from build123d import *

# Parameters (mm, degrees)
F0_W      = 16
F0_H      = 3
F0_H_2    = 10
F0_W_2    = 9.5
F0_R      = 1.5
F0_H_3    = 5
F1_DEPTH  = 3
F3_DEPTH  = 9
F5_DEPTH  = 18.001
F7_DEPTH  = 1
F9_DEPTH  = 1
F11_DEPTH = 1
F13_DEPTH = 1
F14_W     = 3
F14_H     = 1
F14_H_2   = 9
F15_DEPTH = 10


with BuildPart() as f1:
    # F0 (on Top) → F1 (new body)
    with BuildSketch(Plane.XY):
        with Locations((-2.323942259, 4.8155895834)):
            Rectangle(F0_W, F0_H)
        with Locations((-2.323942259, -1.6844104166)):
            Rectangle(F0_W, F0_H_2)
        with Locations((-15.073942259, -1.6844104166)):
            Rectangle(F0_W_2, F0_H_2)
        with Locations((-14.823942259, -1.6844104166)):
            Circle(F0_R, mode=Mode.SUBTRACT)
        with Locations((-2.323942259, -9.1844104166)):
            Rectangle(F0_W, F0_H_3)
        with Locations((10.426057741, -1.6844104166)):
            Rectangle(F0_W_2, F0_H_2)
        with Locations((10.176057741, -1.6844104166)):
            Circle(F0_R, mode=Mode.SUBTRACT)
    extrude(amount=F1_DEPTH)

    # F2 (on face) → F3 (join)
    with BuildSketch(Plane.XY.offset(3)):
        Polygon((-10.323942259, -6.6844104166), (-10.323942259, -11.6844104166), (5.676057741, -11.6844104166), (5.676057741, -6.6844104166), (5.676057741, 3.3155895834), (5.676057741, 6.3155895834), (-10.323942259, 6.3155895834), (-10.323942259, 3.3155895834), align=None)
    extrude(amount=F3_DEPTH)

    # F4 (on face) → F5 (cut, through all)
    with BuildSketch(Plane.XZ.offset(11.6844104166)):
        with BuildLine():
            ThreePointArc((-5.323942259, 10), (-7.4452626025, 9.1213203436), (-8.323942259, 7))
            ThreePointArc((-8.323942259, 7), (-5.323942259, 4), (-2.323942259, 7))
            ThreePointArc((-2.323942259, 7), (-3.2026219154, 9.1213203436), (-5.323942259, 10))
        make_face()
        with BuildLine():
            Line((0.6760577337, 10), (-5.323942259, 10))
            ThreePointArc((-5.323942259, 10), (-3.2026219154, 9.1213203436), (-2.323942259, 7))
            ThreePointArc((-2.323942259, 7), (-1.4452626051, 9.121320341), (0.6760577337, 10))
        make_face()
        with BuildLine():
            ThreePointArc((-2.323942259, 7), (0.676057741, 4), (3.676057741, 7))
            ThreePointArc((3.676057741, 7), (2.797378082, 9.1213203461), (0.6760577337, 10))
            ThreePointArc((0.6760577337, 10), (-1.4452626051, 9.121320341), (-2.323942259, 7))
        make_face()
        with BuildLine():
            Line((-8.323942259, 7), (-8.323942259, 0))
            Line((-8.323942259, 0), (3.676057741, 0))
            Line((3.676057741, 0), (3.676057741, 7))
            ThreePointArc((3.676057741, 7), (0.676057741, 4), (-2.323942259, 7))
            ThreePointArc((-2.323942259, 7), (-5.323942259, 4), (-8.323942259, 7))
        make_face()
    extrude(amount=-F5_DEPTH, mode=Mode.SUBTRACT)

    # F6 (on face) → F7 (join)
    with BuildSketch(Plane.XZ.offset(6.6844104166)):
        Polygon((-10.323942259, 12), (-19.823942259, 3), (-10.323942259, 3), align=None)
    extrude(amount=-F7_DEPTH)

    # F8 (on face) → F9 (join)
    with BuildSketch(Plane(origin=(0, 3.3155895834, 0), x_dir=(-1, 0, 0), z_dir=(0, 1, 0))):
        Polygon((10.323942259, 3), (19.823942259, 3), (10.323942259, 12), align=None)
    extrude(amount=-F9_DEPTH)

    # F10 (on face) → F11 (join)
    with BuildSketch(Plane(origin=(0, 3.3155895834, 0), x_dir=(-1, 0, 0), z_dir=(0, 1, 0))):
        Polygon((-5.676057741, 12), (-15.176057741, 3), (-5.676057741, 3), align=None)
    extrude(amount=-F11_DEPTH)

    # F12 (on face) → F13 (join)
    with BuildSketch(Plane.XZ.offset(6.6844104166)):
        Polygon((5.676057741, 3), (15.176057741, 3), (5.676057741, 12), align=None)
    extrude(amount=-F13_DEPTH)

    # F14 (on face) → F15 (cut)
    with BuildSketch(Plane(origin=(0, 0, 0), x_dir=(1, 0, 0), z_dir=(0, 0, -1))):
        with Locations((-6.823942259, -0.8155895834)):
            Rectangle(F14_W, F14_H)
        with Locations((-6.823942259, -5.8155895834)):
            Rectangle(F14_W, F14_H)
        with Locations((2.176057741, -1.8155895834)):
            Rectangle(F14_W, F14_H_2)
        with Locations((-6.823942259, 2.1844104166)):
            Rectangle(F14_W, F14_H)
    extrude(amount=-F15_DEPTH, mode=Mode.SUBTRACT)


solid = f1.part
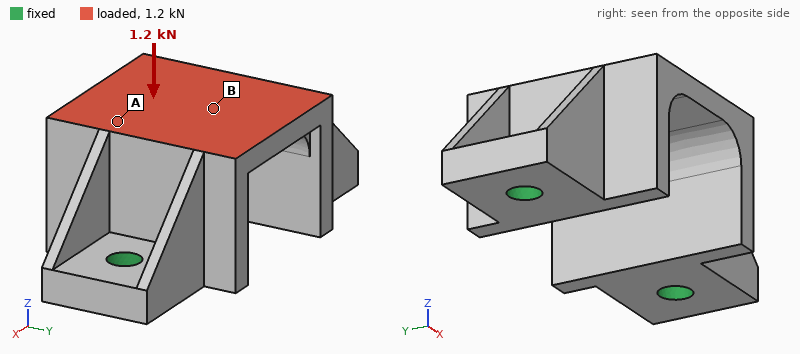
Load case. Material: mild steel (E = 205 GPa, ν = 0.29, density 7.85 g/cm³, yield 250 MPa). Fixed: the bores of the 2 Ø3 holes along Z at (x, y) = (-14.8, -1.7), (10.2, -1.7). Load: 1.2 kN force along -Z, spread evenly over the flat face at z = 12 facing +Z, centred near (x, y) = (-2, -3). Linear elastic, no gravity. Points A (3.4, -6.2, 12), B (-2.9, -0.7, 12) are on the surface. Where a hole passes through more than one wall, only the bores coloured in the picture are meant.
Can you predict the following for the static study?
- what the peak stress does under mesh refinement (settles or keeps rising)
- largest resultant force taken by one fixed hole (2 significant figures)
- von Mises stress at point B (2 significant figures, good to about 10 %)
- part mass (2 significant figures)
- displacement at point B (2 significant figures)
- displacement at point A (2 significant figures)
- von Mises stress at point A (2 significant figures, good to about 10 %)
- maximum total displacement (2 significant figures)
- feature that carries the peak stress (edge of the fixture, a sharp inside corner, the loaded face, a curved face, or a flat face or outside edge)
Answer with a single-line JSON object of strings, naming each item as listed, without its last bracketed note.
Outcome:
{"what the peak stress does under mesh refinement": "keeps rising", "largest resultant force taken by one fixed hole": "710 N", "von Mises stress at point B": "46 MPa", "part mass": "16 g", "displacement at point B": "6.0 µm", "displacement at point A": "5.2 µm", "von Mises stress at point A": "15 MPa", "maximum total displacement": "8.8 µm", "feature that carries the peak stress": "edge of the fixture"}
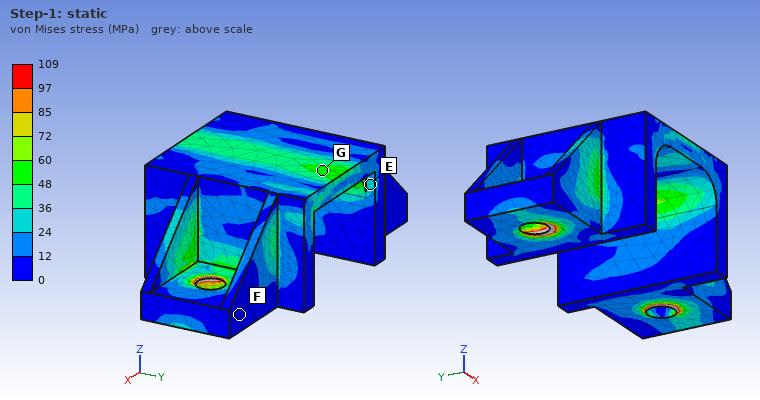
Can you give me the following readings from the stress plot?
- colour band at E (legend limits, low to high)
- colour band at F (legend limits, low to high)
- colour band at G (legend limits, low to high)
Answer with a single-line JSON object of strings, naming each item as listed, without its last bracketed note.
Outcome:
{"colour band at E": "24 to 36 MPa", "colour band at F": "0 to 12 MPa", "colour band at G": "48 to 60 MPa"}
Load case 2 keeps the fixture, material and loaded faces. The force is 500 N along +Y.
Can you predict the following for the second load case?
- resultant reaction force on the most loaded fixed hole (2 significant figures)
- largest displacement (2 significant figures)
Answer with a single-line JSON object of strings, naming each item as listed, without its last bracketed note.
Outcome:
{"resultant reaction force on the most loaded fixed hole": "250 N", "largest displacement": "19 µm"}
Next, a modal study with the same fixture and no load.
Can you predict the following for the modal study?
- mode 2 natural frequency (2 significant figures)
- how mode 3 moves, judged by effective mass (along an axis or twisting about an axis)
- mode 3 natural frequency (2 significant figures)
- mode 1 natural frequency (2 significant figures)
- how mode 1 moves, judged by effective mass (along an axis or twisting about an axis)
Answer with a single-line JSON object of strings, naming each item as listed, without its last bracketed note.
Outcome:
{"mode 2 natural frequency": "17 kHz", "how mode 3 moves, judged by effective mass": "along X", "mode 3 natural frequency": "19 kHz", "mode 1 natural frequency": "11 kHz", "how mode 1 moves, judged by effective mass": "along Y"}
